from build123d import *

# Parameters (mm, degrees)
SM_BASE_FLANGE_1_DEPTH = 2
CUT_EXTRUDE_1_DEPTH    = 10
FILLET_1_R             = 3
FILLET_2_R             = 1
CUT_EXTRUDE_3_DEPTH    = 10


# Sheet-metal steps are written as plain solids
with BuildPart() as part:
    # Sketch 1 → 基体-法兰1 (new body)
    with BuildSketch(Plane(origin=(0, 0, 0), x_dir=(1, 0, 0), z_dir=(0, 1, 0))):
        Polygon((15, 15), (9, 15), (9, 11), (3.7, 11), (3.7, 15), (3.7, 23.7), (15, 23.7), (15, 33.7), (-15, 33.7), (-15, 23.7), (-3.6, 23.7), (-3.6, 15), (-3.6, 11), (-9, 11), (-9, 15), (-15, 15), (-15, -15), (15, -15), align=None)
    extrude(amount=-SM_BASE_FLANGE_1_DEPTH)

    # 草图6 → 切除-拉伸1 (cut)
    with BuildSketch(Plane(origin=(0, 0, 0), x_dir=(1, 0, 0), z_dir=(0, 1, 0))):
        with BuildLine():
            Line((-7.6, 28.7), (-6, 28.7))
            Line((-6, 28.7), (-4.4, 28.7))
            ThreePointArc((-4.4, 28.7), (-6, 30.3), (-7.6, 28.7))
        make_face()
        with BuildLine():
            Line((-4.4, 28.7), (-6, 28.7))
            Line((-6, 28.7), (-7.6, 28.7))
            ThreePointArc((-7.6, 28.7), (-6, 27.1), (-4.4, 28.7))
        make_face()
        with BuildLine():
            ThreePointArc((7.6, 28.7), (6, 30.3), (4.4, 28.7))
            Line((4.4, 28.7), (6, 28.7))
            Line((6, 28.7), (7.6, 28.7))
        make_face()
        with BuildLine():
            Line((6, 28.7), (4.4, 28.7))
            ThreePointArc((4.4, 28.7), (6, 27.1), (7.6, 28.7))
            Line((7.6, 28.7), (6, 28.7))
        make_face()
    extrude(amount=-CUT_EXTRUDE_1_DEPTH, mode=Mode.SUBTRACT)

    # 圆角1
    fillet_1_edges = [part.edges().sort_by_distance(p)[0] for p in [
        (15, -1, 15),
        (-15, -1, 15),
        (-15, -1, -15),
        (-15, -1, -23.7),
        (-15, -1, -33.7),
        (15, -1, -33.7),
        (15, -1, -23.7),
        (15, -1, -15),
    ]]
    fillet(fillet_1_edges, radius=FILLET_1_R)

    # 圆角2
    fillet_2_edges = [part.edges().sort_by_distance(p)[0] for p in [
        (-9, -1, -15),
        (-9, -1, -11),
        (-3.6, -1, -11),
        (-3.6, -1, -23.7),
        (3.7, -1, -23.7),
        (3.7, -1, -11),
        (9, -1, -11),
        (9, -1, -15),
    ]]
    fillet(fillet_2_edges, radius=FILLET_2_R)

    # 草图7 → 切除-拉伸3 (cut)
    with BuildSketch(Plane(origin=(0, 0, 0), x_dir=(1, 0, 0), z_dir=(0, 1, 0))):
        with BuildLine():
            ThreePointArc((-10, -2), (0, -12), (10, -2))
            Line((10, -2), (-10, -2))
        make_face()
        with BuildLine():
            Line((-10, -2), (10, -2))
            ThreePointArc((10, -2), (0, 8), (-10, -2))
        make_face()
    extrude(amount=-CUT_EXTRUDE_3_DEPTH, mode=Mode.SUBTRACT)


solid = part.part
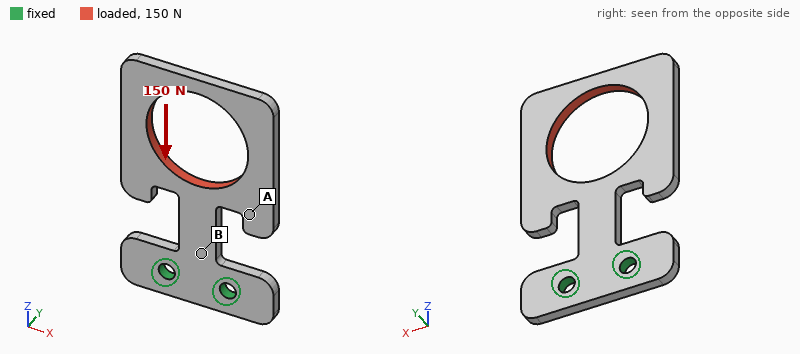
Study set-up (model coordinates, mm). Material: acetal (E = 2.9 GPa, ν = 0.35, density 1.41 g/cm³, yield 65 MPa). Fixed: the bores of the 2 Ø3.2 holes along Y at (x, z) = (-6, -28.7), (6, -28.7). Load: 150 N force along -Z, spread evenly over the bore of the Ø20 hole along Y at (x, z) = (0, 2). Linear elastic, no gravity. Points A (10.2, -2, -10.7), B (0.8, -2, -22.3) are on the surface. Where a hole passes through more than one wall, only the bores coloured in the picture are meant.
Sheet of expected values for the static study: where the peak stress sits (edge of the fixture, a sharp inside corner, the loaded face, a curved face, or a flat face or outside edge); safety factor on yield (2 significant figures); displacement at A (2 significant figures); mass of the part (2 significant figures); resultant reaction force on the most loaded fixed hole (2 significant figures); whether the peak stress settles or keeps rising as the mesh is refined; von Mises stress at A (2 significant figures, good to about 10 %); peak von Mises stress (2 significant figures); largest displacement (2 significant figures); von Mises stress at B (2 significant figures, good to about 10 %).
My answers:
a curved face
0.82
0.25 mm
2.5 g
80 N
settles
3.7 MPa
79 MPa
0.53 mm
7.8 MPa
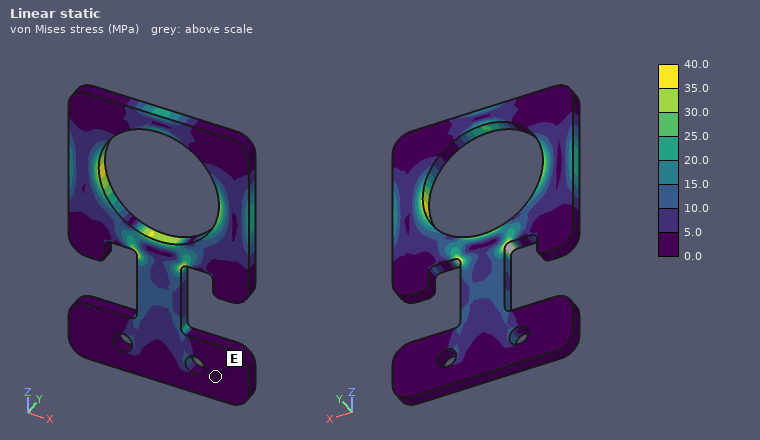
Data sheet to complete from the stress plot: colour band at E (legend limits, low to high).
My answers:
0.0 to 5.0 MPa
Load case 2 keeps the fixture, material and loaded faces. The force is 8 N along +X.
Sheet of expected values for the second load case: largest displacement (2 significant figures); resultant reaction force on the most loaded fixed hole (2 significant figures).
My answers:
0.65 mm
21 N
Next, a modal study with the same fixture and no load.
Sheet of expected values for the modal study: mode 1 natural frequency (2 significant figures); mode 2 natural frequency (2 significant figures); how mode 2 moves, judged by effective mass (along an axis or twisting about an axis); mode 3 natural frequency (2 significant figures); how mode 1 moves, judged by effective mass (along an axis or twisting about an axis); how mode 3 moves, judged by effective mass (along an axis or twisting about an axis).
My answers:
170 Hz
370 Hz
twisting about Z
530 Hz
along Y
along X
